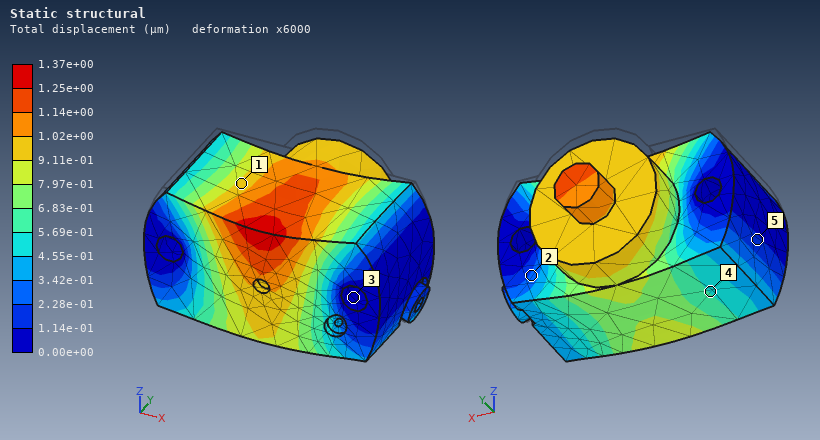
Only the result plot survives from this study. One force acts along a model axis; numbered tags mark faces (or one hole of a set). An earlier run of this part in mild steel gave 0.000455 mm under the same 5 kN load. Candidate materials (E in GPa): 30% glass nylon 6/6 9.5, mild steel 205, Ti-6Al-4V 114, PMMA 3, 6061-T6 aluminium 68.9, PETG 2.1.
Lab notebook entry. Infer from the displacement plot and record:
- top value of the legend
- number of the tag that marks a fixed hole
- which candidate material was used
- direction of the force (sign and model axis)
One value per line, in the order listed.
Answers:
1.37e+00 µm
3
6061-T6 aluminium
-Z
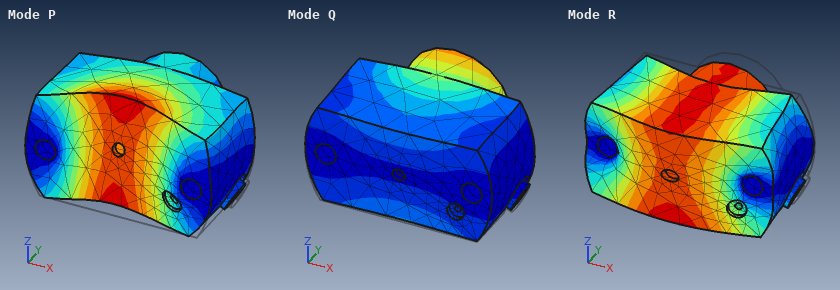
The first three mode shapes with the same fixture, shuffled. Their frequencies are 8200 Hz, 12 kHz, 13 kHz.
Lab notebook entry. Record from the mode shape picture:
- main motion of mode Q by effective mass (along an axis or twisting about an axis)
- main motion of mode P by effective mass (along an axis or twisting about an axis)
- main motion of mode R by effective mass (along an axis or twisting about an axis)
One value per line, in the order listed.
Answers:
along Z
along Z
along Y
